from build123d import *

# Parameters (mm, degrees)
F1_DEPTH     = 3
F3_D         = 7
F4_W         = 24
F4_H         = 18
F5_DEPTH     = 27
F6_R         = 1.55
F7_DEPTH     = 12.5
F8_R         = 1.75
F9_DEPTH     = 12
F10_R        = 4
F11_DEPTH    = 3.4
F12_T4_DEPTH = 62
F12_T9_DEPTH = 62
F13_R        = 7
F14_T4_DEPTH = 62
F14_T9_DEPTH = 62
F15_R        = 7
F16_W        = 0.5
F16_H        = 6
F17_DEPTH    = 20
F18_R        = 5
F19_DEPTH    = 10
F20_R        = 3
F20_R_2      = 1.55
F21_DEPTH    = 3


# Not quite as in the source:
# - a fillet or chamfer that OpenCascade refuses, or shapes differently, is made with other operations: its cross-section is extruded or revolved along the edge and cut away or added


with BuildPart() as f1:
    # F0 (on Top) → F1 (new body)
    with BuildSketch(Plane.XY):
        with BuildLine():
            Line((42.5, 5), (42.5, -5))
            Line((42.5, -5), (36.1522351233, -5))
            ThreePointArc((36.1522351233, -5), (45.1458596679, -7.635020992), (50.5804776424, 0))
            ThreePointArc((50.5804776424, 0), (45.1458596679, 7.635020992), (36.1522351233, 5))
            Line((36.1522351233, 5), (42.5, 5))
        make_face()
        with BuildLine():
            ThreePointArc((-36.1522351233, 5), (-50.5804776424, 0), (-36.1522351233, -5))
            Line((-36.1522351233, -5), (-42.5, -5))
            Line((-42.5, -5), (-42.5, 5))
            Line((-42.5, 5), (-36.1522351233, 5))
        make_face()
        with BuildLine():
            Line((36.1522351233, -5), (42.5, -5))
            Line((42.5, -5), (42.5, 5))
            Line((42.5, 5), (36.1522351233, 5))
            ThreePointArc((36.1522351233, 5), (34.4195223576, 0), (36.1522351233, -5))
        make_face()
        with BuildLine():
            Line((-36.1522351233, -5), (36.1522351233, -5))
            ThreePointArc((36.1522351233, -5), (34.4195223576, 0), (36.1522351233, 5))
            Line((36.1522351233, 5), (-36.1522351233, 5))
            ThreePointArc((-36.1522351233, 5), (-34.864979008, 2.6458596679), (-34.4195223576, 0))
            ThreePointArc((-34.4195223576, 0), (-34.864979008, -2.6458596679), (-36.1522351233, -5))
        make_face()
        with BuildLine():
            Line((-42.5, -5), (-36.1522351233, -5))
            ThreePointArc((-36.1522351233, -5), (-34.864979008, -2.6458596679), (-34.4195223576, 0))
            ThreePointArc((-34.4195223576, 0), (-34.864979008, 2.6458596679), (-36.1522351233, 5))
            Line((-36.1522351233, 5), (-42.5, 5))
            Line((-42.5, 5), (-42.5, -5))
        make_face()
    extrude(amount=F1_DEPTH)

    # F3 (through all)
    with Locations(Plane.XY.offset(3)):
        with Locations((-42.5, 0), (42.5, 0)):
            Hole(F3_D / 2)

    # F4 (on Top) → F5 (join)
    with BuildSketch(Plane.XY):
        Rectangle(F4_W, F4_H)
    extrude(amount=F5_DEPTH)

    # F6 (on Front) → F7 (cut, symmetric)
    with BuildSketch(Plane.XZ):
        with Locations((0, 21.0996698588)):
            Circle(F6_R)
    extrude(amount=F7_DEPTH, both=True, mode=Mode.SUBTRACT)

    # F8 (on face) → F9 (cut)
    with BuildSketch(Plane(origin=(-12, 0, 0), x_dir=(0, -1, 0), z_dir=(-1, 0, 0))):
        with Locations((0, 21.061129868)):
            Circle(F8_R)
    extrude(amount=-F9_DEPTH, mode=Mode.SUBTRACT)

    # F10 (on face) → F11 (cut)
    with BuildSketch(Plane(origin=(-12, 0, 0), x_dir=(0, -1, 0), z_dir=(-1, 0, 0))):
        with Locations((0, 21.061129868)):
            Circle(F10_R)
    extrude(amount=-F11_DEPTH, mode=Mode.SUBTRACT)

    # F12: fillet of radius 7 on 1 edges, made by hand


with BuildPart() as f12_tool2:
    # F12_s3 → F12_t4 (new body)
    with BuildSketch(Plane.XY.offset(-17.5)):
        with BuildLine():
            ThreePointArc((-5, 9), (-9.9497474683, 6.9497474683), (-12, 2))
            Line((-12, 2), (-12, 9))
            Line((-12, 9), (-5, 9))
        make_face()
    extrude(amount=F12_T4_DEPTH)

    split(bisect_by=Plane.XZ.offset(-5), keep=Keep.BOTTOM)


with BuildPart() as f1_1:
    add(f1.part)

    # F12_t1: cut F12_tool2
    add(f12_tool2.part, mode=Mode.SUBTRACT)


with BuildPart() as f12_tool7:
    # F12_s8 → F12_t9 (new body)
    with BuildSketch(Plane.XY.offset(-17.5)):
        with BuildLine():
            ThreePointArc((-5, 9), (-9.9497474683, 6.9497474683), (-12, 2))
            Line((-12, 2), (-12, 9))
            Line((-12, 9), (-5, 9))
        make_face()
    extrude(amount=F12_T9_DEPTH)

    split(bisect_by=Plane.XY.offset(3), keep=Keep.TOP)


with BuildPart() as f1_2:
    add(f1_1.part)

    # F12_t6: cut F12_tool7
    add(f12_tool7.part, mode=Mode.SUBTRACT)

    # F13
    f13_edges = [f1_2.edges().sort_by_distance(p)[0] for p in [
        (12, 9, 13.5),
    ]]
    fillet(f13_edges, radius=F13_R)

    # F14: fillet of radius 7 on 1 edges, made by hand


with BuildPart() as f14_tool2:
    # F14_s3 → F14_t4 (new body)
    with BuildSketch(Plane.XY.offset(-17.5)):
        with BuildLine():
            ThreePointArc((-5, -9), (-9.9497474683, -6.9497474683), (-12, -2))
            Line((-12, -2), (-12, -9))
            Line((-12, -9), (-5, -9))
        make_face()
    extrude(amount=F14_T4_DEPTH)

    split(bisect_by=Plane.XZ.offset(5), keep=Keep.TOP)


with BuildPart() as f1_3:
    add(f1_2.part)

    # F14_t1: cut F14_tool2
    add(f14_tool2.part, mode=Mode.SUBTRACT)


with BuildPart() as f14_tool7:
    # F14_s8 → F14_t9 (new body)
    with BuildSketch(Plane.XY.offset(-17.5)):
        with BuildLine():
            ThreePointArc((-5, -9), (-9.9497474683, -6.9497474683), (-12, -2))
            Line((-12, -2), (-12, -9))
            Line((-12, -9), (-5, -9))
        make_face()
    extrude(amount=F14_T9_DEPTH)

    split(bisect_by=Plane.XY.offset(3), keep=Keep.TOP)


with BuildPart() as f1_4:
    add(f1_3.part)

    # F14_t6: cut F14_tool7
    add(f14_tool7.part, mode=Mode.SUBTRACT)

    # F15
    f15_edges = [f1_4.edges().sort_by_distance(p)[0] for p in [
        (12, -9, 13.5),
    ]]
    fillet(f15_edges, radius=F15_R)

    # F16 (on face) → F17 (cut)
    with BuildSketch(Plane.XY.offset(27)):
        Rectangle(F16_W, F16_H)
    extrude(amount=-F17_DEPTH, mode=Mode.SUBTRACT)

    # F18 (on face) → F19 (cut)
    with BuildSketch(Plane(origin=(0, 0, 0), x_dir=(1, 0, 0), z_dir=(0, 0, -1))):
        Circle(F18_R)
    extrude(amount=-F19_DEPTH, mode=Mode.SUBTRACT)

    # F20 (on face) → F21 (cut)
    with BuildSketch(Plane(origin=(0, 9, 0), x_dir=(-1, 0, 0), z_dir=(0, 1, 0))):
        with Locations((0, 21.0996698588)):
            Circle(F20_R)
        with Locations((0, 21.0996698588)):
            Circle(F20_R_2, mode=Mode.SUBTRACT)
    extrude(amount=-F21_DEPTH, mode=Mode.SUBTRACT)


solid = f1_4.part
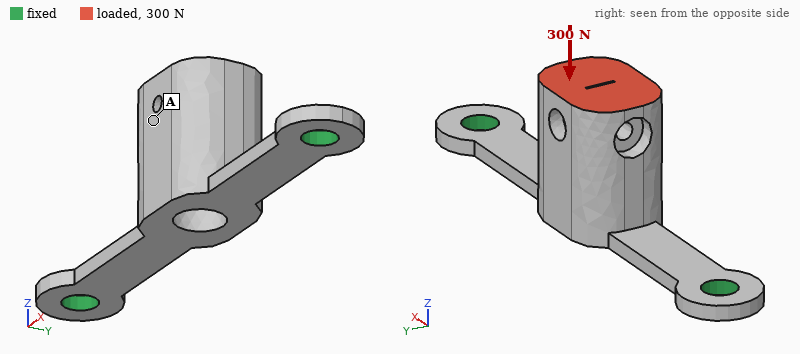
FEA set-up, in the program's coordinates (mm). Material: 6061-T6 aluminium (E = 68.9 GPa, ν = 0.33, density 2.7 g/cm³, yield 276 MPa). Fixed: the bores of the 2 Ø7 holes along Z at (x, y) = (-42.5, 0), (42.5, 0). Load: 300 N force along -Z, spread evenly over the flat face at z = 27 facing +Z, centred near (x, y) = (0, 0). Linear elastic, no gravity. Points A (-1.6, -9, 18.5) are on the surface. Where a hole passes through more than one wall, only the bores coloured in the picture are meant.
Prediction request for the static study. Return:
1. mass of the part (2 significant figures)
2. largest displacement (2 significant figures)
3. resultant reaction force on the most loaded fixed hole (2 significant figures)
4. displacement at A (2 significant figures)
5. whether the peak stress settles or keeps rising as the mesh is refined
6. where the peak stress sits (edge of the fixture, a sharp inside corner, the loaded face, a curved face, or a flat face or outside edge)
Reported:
31 g
0.19 mm
180 N
0.19 mm
keeps rising
edge of the fixture
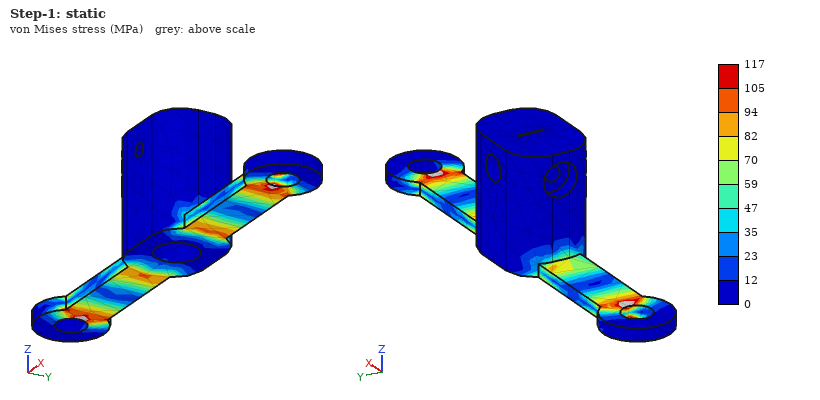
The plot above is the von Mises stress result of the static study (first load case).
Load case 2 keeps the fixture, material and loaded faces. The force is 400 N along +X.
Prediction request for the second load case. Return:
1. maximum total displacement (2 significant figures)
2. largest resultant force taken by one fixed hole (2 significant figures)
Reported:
0.27 mm
270 N
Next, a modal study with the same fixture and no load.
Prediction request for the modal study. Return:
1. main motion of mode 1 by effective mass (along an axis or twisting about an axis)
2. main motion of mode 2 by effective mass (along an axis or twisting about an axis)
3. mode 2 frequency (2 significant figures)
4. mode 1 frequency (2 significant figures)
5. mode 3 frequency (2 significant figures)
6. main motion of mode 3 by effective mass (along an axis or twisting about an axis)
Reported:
along Y
along Z
1200 Hz
790 Hz
2000 Hz
along X
